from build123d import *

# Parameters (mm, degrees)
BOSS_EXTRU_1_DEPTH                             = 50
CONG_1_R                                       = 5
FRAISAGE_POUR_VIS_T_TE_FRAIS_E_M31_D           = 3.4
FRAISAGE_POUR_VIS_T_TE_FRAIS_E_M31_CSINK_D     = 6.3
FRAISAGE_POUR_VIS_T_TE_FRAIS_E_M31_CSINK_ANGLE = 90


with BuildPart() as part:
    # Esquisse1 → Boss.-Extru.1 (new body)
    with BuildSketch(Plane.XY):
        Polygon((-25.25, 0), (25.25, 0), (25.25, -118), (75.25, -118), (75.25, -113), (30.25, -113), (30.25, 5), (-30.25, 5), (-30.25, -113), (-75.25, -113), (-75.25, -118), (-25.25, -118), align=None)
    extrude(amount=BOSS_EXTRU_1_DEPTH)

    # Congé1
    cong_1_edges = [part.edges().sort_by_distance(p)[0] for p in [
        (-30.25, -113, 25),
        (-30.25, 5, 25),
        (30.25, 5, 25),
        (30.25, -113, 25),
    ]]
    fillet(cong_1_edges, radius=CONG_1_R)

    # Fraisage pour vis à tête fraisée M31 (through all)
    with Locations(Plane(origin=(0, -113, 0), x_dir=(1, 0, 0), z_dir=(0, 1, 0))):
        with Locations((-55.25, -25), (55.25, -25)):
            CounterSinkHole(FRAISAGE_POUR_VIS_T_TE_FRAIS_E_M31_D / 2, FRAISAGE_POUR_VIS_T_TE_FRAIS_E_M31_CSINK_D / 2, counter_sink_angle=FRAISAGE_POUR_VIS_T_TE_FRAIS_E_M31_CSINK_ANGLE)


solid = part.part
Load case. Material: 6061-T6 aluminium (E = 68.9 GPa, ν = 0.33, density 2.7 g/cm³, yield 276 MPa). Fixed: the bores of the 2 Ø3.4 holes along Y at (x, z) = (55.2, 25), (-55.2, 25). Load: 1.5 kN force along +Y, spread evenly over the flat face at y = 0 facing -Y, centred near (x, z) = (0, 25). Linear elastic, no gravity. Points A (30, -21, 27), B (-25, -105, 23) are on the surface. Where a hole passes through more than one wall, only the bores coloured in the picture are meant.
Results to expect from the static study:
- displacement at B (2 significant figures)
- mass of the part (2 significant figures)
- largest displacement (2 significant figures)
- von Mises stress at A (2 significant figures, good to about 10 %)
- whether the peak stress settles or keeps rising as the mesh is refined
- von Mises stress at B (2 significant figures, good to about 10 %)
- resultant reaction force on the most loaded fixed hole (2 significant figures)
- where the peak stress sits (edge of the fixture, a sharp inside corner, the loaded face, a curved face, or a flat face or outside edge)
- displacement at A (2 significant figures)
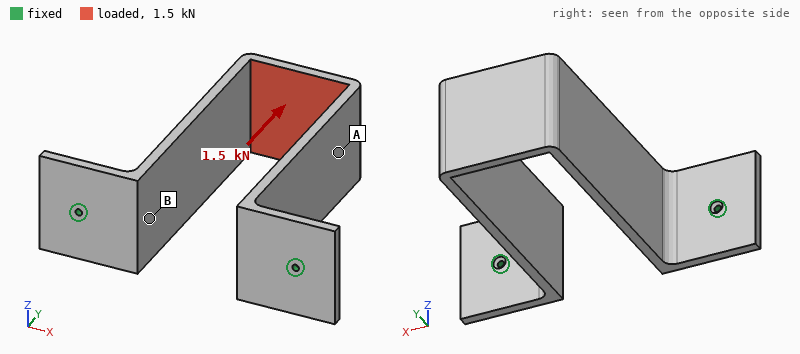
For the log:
0.18 mm
260 g
0.21 mm
9.5 MPa
keeps rising
31 MPa
760 N
edge of the fixture
0.17 mm
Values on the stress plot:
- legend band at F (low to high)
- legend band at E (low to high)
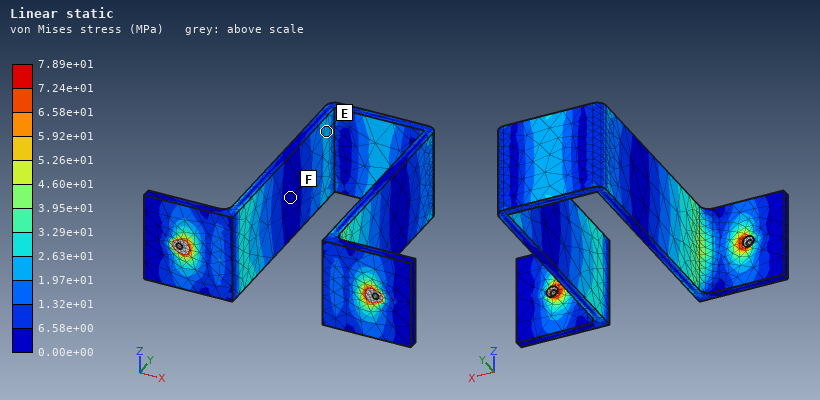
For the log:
0.00e+00 to 6.58e+00 MPa
1.97e+01 to 2.63e+01 MPa
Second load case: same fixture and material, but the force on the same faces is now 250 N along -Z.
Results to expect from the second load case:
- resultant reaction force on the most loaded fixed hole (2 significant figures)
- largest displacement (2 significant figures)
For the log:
130 N
1.3 mm
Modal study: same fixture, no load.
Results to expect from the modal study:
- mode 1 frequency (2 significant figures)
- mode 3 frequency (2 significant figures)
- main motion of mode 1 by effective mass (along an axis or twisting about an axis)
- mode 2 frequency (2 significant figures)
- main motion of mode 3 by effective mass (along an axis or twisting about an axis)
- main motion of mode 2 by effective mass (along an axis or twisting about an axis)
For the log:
230 Hz
720 Hz
along Z
330 Hz
twisting about Y
along X
